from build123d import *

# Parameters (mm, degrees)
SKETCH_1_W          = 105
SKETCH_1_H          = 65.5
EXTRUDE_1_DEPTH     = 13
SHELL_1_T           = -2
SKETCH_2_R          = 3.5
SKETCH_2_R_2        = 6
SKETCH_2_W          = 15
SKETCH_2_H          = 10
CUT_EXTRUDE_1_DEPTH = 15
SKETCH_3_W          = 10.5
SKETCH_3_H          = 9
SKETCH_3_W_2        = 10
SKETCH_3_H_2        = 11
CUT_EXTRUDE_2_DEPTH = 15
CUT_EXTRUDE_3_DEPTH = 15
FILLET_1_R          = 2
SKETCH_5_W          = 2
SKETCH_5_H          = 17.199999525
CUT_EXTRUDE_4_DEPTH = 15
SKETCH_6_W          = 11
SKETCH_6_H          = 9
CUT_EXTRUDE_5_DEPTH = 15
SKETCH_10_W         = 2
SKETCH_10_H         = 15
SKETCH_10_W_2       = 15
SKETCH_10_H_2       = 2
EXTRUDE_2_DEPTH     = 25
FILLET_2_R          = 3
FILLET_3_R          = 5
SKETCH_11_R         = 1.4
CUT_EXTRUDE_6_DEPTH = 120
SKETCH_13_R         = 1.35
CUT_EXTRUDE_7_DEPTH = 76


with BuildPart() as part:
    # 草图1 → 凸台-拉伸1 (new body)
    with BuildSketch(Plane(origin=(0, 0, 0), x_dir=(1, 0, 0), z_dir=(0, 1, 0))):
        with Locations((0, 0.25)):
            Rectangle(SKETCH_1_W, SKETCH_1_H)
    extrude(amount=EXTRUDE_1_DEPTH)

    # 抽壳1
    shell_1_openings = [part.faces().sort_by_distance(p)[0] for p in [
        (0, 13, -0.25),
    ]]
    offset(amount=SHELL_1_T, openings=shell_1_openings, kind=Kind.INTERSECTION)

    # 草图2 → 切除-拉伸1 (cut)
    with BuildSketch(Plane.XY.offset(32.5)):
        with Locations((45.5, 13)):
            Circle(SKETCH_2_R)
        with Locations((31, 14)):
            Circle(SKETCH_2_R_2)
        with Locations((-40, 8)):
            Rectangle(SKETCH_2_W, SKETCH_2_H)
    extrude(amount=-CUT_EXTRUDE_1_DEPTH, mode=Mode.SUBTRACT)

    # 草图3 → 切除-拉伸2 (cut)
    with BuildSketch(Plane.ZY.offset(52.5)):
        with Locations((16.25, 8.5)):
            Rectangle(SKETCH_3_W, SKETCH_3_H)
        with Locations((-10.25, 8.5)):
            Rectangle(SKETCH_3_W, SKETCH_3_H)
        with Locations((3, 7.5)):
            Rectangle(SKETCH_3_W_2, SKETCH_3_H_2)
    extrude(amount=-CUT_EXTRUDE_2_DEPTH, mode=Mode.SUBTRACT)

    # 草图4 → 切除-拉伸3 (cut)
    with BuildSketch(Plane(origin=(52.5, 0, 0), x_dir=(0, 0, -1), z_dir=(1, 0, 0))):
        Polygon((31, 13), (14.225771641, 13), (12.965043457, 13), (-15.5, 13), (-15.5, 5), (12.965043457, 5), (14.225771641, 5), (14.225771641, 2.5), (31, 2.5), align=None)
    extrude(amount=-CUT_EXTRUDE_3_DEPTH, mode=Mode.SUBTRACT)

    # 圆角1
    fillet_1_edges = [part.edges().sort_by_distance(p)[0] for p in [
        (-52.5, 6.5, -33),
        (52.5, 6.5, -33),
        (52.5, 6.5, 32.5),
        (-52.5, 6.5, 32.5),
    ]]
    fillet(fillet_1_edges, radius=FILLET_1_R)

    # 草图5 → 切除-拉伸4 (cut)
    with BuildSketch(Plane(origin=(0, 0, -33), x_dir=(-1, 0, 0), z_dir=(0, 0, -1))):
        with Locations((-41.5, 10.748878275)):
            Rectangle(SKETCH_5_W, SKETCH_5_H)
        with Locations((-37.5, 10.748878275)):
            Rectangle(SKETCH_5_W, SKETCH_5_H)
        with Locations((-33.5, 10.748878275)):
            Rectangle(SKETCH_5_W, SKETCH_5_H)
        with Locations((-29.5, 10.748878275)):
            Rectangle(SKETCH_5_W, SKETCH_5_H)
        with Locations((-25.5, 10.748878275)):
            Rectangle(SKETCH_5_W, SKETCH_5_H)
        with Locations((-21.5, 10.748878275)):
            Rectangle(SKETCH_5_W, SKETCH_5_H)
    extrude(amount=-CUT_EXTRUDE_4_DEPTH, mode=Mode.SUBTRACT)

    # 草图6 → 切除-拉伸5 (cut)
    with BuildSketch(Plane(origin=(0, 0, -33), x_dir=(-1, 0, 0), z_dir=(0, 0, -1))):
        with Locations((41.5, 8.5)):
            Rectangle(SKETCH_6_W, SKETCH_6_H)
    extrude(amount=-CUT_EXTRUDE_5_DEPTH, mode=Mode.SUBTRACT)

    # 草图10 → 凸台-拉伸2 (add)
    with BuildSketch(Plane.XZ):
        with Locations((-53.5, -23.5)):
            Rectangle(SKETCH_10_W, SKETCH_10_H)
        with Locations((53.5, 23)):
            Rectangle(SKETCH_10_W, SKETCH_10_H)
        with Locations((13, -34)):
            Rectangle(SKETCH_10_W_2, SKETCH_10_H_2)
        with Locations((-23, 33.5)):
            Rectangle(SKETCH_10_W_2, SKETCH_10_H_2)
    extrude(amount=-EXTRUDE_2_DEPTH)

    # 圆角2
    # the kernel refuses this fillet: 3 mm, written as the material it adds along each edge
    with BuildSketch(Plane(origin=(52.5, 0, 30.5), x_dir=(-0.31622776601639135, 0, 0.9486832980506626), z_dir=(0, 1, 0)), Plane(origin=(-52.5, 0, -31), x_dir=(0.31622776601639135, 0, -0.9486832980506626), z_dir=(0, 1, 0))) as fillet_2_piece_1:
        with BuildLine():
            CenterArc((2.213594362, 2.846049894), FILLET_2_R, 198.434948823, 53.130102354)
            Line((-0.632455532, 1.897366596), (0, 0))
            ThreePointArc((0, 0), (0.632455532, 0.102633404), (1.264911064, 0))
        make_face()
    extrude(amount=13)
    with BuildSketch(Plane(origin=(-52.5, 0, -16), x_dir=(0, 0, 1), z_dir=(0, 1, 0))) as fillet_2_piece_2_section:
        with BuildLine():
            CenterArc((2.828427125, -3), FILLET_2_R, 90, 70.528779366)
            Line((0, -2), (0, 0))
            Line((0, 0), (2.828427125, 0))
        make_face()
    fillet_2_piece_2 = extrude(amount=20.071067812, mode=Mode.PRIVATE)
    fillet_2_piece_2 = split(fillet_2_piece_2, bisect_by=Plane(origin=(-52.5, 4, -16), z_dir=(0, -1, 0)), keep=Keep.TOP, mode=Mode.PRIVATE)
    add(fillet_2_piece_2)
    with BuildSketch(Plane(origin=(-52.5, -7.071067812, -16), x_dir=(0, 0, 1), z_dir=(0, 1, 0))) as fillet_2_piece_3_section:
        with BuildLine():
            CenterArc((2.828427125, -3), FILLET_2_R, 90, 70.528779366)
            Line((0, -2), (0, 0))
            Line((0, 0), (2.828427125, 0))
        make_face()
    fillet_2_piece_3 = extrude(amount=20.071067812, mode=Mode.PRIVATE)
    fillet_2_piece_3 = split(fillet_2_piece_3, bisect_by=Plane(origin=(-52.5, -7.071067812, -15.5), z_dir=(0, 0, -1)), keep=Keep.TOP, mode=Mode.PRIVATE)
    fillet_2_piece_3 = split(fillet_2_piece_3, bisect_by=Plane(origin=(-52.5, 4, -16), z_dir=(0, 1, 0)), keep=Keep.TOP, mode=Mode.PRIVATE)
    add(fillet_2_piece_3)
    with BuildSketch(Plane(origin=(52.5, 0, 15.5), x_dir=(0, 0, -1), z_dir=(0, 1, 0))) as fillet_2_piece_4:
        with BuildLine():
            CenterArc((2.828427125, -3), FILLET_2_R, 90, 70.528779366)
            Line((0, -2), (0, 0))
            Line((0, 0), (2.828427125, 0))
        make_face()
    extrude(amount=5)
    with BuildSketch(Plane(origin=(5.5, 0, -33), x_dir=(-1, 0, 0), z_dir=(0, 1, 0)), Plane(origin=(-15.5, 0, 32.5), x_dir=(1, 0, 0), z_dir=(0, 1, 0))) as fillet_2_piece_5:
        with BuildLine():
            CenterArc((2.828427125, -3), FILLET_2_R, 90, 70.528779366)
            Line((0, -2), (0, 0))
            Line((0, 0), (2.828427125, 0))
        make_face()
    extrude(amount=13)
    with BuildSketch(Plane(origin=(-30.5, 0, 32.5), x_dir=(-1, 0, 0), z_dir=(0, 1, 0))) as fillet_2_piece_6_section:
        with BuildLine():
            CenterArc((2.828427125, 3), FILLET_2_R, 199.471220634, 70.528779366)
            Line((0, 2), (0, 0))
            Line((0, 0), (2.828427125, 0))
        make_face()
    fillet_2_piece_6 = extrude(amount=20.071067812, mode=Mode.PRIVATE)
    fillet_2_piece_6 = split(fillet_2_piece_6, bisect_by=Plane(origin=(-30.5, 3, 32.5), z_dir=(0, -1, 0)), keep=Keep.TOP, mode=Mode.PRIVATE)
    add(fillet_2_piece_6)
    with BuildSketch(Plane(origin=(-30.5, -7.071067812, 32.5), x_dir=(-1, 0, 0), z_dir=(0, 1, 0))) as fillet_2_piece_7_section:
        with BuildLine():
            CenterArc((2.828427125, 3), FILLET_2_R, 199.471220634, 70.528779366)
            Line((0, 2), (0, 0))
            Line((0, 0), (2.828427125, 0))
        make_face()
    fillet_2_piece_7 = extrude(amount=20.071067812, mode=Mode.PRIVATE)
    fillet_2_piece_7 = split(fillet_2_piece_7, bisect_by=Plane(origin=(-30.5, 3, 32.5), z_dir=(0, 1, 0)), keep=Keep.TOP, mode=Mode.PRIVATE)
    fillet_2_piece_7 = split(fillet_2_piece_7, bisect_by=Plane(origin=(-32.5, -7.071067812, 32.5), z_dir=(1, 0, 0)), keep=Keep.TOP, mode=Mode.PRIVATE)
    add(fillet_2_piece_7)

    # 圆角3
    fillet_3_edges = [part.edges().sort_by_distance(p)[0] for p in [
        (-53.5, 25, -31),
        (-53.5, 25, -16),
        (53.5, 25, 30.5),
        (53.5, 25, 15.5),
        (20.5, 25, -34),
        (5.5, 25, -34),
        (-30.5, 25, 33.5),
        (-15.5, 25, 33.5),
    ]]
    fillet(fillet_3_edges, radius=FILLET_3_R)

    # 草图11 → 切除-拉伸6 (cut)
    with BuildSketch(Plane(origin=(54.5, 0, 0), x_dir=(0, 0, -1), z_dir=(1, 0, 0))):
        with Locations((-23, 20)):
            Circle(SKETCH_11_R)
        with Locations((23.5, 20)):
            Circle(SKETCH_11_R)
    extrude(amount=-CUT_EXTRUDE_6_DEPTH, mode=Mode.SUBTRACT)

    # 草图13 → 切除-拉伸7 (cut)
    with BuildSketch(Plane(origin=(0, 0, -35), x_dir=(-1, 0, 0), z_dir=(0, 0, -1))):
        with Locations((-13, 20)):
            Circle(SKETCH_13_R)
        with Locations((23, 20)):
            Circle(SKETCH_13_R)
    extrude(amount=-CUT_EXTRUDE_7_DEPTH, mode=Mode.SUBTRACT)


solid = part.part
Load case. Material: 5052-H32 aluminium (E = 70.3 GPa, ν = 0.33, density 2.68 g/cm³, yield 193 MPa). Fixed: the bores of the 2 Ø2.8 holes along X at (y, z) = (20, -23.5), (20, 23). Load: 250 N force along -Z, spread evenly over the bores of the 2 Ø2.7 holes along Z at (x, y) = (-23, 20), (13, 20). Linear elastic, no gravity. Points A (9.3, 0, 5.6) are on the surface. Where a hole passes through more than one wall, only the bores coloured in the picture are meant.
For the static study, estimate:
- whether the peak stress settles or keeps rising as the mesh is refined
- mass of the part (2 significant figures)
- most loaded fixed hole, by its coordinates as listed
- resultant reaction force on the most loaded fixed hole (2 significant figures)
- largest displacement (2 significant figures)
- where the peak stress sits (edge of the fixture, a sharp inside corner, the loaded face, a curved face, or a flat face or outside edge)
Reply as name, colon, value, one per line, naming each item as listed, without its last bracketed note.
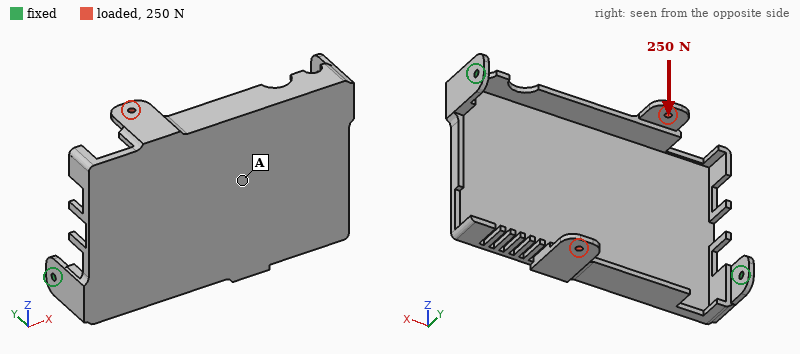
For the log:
whether the peak stress settles or keeps rising as the mesh is refined: keeps rising
mass of the part: 58 g
most loaded fixed hole, by its coordinates as listed: (20, -23.5)
resultant reaction force on the most loaded fixed hole: 140 N
largest displacement: 1.0 mm
where the peak stress sits: a sharp inside corner
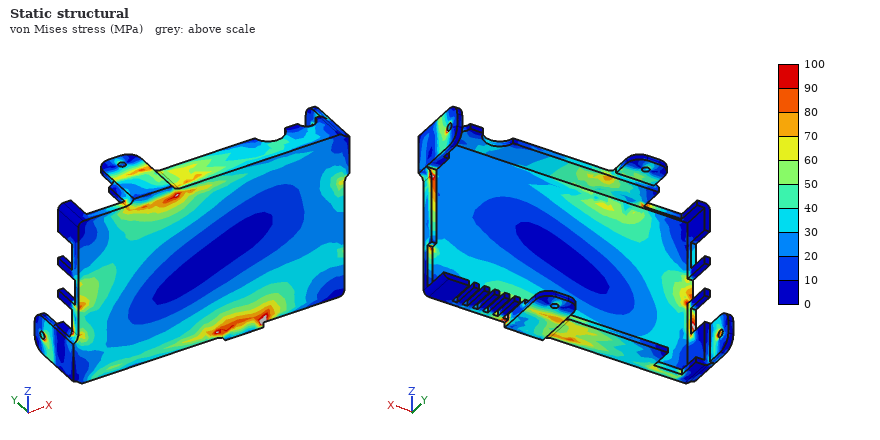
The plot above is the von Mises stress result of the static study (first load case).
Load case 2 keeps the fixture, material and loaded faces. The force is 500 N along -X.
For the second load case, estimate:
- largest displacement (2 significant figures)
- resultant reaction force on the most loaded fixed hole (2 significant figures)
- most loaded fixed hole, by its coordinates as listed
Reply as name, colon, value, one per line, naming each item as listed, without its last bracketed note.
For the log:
largest displacement: 0.66 mm
resultant reaction force on the most loaded fixed hole: 320 N
most loaded fixed hole, by its coordinates as listed: (20, 23)
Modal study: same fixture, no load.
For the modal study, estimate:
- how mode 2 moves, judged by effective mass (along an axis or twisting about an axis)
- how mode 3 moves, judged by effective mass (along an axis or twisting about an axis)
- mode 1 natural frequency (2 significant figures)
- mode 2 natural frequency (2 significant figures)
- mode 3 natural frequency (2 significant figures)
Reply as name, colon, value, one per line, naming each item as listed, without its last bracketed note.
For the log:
how mode 2 moves, judged by effective mass: along Y
how mode 3 moves, judged by effective mass: along X
mode 1 natural frequency: 500 Hz
mode 2 natural frequency: 650 Hz
mode 3 natural frequency: 1200 Hz
